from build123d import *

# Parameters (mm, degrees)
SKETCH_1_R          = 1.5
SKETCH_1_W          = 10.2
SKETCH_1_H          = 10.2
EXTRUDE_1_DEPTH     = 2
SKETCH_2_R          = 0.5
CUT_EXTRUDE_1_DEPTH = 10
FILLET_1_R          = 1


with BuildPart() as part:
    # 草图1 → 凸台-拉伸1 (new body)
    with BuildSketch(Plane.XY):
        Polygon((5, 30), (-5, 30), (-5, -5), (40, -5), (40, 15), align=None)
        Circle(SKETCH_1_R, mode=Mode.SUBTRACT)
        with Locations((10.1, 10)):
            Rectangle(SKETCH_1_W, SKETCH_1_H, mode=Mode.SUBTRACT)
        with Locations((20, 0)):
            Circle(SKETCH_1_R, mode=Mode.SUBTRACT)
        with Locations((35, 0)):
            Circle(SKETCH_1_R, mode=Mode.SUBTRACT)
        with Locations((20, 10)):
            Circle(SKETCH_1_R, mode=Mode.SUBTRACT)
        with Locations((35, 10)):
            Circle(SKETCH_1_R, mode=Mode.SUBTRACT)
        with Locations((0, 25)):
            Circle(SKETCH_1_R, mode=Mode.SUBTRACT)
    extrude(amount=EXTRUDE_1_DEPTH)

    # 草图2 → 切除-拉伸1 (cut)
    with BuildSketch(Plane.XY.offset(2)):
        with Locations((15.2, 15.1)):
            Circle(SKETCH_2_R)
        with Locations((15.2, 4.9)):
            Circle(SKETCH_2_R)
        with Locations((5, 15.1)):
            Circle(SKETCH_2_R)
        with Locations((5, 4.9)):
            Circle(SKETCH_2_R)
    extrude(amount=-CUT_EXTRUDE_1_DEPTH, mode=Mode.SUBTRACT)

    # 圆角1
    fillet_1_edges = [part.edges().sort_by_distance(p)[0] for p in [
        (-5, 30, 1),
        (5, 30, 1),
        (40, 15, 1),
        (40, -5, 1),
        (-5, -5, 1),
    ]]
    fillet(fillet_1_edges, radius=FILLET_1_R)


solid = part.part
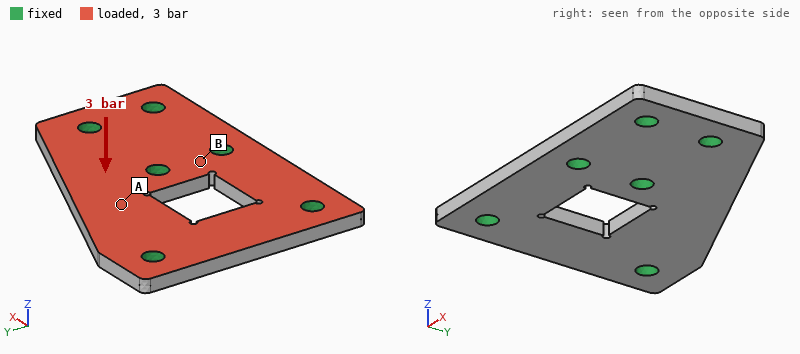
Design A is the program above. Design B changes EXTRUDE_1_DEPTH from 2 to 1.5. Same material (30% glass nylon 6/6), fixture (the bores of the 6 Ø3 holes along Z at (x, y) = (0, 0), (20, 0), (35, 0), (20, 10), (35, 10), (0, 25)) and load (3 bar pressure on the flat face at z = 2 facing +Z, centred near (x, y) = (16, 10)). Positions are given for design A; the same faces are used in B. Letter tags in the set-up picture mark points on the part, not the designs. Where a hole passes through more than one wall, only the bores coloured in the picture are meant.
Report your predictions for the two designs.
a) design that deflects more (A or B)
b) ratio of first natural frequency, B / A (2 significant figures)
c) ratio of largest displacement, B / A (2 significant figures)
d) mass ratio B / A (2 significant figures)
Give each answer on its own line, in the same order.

B
0.78
2.2
0.75
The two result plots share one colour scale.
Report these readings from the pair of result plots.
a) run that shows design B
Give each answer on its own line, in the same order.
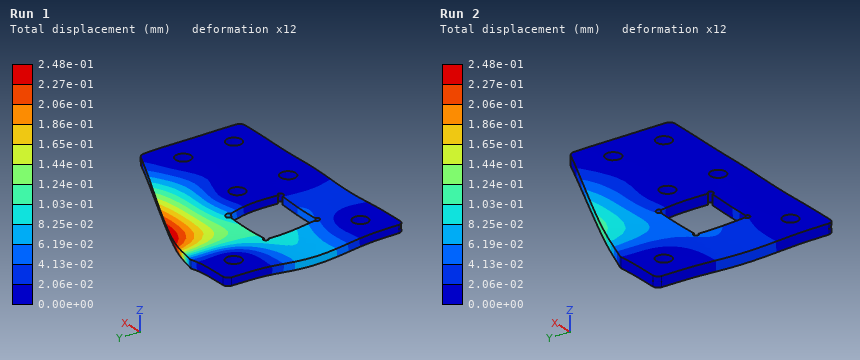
Run 1
